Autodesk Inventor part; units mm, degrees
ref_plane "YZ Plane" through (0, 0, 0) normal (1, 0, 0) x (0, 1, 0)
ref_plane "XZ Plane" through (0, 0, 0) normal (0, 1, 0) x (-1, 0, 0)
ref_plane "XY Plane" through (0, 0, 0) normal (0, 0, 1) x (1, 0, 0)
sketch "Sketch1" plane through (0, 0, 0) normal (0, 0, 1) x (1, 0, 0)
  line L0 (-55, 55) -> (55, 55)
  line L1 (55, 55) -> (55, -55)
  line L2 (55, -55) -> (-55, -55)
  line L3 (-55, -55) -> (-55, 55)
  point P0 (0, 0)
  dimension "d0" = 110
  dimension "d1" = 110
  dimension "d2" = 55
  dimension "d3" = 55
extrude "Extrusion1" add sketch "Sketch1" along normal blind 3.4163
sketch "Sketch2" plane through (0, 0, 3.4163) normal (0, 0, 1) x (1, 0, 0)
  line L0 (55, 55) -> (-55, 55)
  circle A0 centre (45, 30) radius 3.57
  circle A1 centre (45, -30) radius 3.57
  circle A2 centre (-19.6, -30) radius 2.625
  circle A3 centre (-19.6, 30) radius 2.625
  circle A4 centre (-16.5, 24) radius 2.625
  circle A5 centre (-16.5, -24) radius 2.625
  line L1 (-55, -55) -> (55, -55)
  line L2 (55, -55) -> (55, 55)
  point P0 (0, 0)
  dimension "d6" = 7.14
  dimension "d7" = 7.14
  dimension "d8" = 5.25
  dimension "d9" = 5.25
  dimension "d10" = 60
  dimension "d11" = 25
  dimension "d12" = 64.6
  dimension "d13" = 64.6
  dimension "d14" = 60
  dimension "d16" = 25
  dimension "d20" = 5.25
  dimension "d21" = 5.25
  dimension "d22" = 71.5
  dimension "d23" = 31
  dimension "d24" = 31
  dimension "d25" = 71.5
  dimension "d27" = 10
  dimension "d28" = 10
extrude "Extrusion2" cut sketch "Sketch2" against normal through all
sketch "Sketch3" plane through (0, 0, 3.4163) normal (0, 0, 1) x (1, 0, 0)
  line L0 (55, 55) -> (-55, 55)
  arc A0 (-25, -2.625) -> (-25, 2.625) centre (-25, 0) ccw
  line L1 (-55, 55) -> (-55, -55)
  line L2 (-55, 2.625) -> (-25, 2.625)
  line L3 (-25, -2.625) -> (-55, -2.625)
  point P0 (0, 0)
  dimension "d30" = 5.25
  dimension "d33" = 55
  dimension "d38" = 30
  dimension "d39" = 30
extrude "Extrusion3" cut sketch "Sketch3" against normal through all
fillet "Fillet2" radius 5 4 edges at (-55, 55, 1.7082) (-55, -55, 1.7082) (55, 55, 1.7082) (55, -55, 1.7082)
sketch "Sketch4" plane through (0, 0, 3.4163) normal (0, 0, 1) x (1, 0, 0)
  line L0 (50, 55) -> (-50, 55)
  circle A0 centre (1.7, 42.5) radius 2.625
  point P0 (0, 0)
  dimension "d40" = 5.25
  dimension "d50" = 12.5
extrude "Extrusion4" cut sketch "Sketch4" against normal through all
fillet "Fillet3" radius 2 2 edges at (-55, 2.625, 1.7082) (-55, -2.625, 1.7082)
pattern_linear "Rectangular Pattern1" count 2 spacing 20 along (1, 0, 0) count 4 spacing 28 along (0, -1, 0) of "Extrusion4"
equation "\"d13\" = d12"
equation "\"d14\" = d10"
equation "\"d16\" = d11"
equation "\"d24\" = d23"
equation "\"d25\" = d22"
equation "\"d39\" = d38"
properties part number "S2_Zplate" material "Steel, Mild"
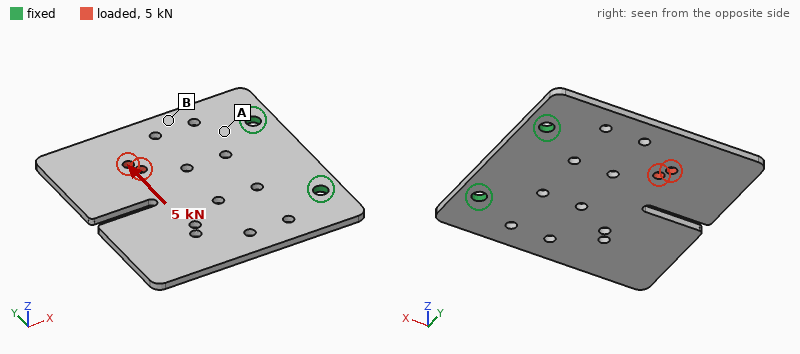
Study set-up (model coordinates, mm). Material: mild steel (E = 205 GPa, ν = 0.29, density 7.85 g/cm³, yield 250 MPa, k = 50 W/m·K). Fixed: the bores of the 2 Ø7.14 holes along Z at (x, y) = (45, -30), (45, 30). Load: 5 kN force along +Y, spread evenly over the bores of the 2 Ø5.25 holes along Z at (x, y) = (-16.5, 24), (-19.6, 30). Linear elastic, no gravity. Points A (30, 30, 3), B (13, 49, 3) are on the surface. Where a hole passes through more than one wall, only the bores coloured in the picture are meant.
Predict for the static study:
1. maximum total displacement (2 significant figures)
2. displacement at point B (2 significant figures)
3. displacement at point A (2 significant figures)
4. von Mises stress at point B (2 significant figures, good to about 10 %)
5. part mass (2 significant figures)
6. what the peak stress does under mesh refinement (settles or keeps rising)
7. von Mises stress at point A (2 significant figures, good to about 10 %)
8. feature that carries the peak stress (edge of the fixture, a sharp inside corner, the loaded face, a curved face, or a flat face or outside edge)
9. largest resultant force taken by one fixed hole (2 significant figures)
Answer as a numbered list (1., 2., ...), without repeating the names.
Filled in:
1. 50 µm
2. 23 µm
3. 8.0 µm
4. 21 MPa
5. 310 g
6. keeps rising
7. 51 MPa
8. edge of the fixture
9. 5.5 kN
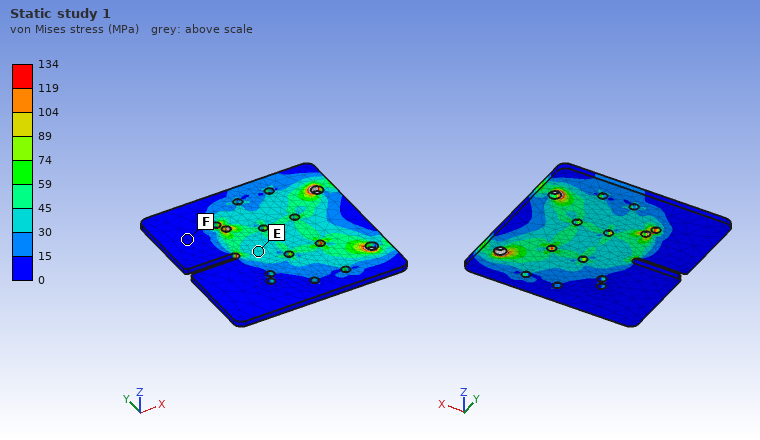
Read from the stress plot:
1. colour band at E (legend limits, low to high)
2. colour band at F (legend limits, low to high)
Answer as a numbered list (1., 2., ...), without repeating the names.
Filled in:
1. 30 to 45 MPa
2. 0 to 15 MPa
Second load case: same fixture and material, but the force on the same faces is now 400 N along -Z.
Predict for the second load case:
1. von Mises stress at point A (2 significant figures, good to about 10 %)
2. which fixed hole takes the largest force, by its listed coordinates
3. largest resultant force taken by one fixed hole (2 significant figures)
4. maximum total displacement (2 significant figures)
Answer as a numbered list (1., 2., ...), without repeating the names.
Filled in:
1. 120 MPa
2. (45, 30)
3. 350 N
4. 1.2 mm
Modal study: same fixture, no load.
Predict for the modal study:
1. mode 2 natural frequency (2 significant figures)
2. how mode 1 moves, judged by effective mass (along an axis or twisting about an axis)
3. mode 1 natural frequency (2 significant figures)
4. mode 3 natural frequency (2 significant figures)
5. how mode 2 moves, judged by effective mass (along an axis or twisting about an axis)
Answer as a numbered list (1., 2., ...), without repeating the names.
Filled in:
1. 550 Hz
2. along Z
3. 280 Hz
4. 1400 Hz
5. twisting about X
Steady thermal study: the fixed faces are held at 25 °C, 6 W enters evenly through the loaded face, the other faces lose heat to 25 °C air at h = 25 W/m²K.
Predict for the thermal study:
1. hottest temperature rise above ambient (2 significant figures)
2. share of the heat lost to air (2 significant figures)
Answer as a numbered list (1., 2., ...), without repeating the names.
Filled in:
1. 26 K
2. 66 %
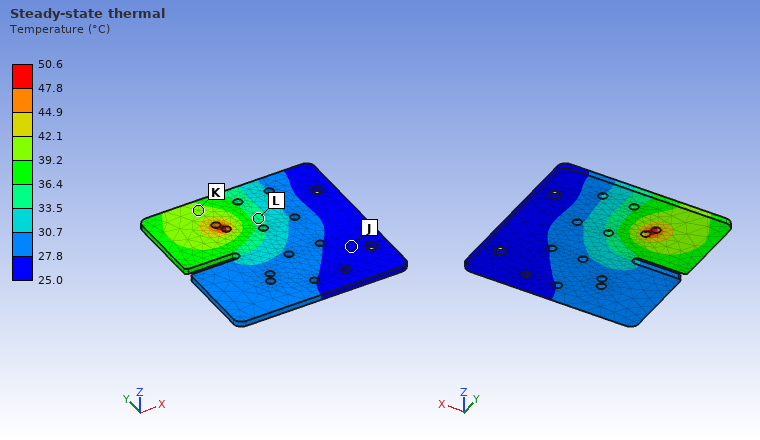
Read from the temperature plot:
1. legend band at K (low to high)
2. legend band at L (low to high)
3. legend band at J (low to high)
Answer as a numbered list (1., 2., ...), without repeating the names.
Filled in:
1. 39.2 to 42.1 °C
2. 33.5 to 36.4 °C
3. 25.0 to 27.8 °C
